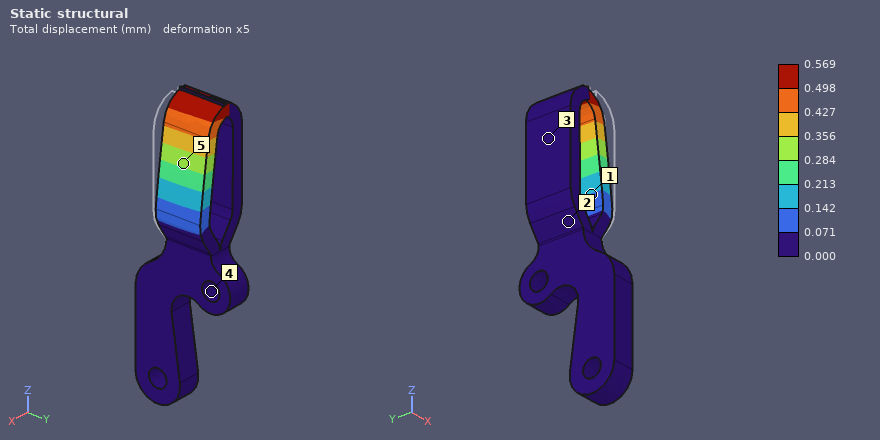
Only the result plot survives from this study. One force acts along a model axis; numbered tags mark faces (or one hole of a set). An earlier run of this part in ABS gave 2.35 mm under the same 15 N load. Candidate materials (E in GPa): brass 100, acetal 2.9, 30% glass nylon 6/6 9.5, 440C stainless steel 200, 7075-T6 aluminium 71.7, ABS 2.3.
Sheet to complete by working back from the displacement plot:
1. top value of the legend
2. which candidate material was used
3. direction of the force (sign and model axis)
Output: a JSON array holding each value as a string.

["0.569 mm", "30% glass nylon 6/6", "-X"]
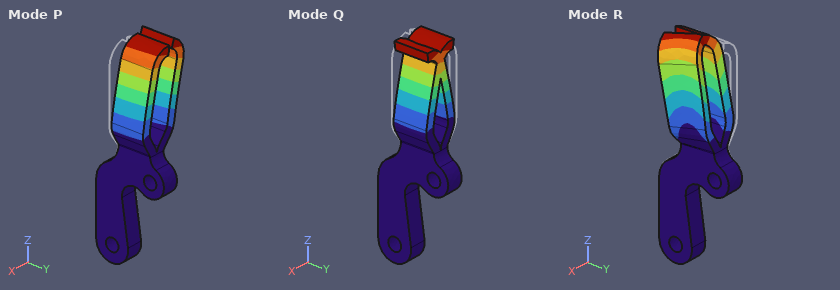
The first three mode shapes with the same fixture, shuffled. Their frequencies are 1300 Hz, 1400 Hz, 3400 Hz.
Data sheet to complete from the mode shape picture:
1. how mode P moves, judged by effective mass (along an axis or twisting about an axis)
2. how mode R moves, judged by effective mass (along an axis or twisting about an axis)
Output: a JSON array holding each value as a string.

["along X", "along Y"]
